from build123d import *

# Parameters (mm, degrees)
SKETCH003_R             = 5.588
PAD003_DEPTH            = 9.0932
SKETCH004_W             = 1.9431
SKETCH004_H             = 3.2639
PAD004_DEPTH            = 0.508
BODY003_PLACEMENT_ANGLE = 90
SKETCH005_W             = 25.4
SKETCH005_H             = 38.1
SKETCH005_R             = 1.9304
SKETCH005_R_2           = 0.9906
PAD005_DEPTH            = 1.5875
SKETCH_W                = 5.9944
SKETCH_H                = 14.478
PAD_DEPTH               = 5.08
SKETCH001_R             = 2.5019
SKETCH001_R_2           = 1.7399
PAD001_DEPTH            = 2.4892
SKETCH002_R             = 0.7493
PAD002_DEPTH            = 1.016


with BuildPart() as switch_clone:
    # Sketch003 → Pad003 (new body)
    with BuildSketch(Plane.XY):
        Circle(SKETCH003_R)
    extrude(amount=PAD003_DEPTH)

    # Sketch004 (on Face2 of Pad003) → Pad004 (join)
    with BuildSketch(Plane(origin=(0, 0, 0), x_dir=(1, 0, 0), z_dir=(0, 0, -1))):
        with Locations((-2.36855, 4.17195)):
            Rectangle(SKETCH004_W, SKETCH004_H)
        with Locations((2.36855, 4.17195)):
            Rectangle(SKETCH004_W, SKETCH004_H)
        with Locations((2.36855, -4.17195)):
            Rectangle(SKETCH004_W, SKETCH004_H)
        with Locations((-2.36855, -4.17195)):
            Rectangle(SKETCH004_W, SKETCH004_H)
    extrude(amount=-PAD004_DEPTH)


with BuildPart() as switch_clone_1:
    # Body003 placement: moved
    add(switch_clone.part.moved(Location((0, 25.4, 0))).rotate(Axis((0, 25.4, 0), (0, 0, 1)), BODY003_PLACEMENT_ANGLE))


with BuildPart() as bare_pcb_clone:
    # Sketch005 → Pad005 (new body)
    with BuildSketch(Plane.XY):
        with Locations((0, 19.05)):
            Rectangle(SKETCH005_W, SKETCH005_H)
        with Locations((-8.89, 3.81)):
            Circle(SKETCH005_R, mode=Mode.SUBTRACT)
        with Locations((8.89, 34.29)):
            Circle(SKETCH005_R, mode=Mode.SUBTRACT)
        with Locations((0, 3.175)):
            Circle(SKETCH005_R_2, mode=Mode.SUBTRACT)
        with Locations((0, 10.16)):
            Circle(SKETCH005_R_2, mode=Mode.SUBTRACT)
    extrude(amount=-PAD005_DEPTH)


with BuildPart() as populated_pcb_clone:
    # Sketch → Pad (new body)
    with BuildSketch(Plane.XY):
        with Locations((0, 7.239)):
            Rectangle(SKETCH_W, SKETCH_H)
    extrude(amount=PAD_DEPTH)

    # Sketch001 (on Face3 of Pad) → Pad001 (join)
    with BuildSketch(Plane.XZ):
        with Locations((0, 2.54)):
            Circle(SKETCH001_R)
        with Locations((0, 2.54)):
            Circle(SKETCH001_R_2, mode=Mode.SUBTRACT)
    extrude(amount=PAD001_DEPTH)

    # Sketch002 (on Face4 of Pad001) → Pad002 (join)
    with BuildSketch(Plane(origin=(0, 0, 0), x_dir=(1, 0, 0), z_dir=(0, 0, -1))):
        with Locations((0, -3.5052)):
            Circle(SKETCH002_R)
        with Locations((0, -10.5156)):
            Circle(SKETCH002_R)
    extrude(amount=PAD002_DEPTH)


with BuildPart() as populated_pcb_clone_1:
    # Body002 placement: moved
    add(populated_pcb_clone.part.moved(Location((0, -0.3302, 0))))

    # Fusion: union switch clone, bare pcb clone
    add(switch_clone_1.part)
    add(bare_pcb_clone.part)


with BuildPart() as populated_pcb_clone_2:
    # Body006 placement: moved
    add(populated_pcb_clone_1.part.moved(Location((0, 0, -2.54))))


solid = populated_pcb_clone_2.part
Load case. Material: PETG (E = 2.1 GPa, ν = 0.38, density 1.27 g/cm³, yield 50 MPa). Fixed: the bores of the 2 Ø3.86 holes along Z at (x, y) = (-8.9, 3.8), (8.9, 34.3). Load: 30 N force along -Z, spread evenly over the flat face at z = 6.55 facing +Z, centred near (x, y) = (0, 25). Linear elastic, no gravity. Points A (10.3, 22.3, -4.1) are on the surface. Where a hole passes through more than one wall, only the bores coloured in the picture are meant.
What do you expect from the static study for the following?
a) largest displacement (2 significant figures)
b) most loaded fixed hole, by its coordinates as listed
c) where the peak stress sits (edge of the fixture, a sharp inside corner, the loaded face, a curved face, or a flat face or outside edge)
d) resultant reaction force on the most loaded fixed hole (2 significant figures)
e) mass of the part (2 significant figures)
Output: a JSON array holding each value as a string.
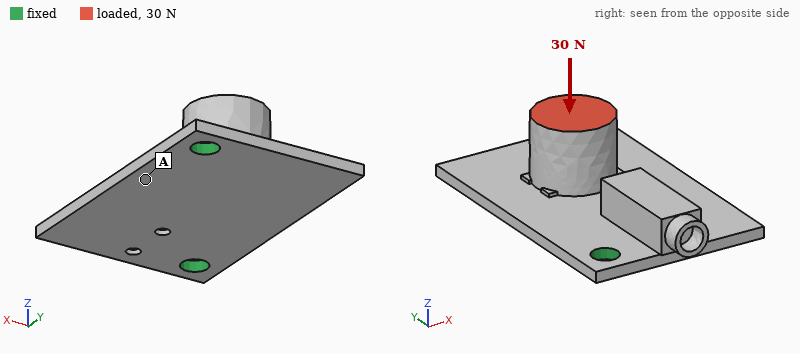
["0.47 mm", "(8.9, 34.3)", "a flat face or outside edge", "21 N", "3.6 g"]
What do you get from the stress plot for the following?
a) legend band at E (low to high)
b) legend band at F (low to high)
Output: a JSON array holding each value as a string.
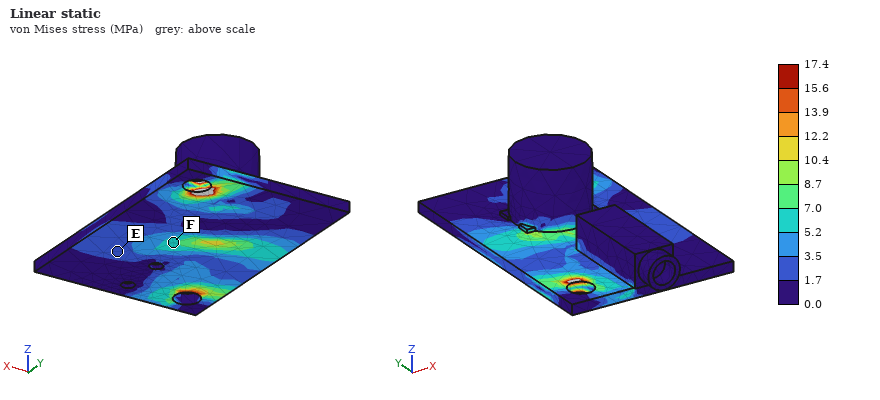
["1.7 to 3.5 MPa", "5.2 to 7.0 MPa"]
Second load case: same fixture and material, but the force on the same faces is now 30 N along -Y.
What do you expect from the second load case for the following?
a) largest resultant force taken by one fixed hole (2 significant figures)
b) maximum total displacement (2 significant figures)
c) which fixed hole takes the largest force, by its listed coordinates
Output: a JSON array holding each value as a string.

["20 N", "0.57 mm", "(8.9, 34.3)"]
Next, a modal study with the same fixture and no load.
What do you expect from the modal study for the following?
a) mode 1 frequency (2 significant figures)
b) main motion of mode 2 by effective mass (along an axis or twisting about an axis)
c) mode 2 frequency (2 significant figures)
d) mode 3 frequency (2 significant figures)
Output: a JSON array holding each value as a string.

["830 Hz", "along Z", "1100 Hz", "1900 Hz"]
